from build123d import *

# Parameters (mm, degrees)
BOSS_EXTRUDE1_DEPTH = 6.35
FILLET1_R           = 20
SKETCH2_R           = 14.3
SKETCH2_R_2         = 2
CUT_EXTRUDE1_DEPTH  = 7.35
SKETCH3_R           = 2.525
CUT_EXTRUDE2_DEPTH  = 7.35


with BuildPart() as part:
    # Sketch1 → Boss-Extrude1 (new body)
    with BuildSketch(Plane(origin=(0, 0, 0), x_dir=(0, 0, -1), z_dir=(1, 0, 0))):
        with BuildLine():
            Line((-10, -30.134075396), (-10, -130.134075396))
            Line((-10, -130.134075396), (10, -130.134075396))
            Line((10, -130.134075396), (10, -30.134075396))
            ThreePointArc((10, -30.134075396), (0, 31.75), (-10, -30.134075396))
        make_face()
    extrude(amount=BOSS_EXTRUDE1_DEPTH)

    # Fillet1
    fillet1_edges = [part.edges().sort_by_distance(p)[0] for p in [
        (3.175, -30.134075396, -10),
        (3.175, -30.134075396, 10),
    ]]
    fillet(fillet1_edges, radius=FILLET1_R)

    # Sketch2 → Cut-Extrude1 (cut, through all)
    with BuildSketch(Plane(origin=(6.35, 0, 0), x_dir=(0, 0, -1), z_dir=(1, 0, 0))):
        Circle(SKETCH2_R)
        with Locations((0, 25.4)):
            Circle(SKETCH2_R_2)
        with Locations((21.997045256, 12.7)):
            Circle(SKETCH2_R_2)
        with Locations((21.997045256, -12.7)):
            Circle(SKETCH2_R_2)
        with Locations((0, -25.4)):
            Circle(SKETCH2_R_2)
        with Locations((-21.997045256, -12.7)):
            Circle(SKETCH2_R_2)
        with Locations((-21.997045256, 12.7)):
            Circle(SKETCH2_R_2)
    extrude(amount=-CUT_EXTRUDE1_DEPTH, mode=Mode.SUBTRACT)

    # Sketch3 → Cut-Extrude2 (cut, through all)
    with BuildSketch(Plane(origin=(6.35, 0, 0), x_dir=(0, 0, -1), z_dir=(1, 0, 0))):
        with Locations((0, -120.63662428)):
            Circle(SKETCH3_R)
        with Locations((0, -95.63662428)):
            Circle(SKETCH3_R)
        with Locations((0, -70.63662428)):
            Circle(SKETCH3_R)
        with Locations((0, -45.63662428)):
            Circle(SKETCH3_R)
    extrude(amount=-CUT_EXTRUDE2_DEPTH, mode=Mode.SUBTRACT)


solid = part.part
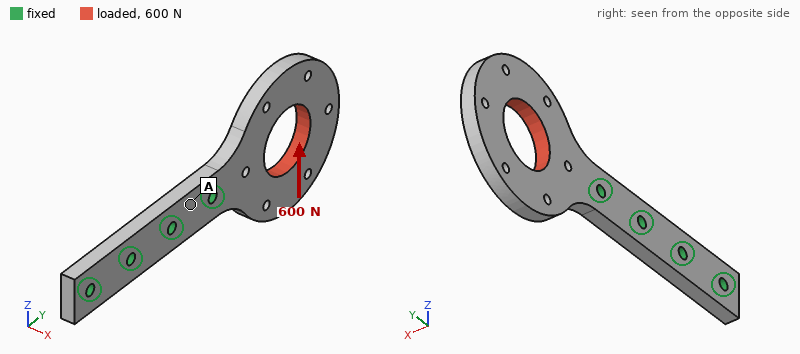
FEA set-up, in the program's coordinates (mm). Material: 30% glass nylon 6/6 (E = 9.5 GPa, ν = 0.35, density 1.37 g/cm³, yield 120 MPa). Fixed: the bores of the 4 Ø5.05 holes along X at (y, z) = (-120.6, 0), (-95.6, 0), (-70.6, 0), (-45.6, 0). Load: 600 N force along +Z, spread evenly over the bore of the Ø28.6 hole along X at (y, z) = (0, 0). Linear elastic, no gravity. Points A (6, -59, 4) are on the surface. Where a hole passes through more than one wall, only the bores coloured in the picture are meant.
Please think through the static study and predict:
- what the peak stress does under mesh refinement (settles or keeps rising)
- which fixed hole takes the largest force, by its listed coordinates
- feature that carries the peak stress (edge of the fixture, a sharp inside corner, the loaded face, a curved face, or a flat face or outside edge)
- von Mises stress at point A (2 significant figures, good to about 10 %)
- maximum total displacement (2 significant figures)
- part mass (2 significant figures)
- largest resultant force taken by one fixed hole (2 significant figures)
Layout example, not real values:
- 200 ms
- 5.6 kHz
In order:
- keeps rising
- (-45.6, 0)
- edge of the fixture
- 14 MPa
- 1.2 mm
- 38 g
- 1.3 kN
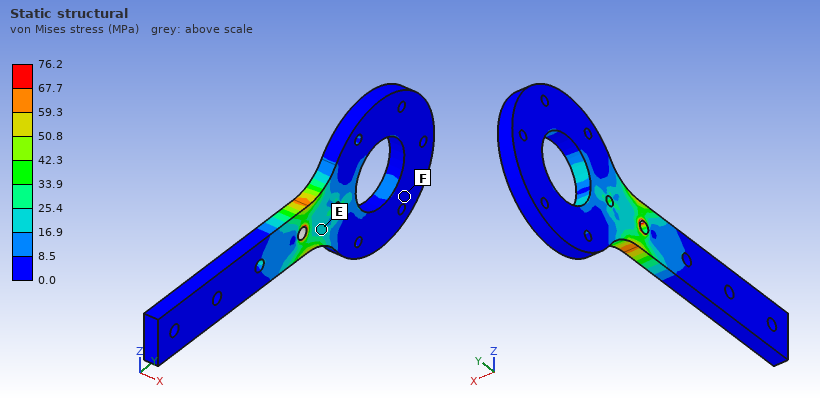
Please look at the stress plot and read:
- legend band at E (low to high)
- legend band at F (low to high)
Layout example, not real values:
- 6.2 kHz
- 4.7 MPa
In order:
- 16.9 to 25.4 MPa
- 0.0 to 8.5 MPa
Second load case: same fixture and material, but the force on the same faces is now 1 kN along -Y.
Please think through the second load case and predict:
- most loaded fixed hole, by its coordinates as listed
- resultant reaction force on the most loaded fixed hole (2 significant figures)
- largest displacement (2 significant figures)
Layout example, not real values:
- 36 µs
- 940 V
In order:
- (-45.6, 0)
- 880 N
- 59 µm
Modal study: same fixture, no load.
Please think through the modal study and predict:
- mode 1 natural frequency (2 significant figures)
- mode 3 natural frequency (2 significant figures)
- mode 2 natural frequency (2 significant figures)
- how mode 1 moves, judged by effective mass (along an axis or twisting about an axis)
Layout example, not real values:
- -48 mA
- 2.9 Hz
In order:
- 360 Hz
- 870 Hz
- 840 Hz
- along X
